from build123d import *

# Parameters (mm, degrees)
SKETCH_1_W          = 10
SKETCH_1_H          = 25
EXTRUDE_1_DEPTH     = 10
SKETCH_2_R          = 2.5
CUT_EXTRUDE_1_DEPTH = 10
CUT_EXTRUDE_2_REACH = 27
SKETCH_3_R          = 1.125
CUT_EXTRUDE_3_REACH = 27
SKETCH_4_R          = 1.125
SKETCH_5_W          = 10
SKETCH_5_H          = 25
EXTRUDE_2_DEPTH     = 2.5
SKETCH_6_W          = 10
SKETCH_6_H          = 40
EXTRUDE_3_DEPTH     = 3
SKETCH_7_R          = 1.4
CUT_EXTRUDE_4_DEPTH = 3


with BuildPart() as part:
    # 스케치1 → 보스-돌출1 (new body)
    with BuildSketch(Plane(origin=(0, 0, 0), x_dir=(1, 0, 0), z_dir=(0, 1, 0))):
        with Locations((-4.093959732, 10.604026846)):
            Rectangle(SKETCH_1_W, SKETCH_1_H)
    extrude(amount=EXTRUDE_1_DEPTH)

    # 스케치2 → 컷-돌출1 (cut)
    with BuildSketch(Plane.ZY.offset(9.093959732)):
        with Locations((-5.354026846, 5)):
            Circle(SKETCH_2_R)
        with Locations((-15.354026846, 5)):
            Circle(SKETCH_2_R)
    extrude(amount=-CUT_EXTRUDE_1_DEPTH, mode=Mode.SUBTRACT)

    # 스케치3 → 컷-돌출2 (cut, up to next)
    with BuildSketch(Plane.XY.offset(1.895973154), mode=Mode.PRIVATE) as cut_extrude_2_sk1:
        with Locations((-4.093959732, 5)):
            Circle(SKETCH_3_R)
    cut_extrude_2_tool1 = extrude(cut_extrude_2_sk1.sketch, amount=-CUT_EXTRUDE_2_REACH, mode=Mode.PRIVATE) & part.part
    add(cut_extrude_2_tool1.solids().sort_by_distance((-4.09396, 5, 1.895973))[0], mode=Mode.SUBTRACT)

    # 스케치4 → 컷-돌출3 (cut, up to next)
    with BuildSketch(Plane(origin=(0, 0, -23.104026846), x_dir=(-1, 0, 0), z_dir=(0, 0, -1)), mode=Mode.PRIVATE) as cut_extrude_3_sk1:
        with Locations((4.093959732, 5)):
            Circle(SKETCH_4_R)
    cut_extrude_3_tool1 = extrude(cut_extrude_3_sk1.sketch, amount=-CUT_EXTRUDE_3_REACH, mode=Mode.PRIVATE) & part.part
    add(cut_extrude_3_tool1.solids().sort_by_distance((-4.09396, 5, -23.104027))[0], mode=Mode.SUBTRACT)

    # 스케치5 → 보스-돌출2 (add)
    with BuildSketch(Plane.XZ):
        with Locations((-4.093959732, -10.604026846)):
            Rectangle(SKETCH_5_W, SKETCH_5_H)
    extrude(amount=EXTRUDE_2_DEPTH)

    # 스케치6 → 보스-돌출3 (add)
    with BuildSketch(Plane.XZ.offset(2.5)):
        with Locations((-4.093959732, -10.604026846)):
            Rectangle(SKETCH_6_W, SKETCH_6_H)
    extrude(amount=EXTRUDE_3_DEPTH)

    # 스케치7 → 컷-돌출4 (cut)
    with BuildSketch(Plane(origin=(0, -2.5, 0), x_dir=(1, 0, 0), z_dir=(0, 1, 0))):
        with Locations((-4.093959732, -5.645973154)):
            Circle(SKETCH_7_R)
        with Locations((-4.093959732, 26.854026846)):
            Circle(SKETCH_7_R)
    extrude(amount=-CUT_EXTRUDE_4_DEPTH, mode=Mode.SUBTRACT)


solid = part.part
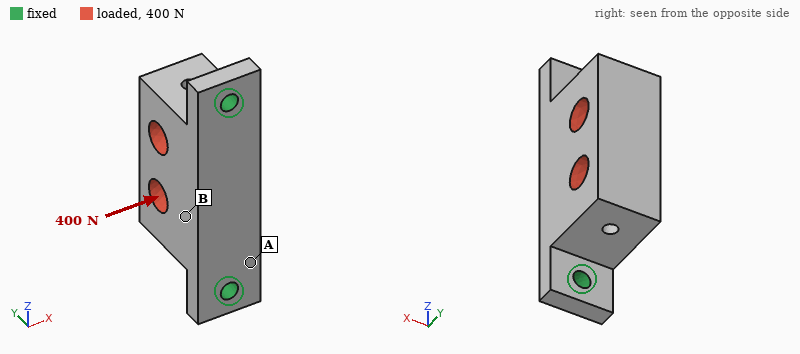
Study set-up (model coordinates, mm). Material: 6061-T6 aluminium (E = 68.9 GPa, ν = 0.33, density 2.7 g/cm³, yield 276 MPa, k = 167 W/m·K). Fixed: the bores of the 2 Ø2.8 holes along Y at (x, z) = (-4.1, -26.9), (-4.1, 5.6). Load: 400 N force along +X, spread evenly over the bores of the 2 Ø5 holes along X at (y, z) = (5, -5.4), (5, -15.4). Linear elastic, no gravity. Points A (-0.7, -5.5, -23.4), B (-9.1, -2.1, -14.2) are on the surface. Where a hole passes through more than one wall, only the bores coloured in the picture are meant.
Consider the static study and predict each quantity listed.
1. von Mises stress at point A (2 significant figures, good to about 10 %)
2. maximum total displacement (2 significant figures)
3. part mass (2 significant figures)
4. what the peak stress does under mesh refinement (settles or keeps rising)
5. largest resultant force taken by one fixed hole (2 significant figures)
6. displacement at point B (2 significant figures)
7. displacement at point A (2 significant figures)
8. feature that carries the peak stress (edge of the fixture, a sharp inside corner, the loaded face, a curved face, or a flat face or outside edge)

38 MPa
53 µm
10 g
keeps rising
200 N
19 µm
8.6 µm
edge of the fixture
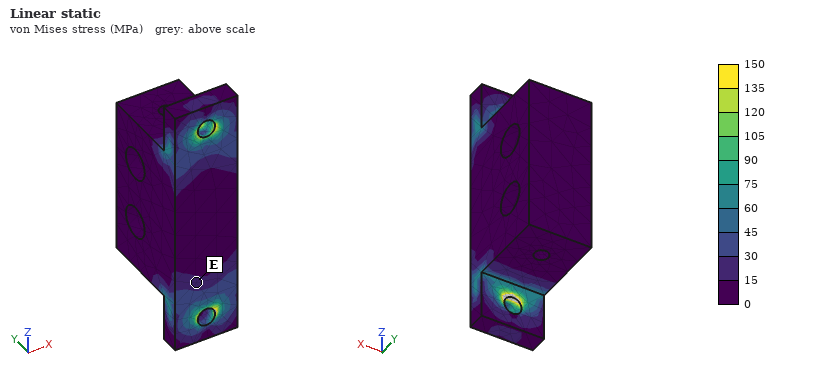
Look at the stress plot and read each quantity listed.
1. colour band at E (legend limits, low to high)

15 to 30 MPa
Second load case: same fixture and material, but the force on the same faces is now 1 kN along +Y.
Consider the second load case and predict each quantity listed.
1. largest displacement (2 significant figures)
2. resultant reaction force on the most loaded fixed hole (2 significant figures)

10 µm
590 N
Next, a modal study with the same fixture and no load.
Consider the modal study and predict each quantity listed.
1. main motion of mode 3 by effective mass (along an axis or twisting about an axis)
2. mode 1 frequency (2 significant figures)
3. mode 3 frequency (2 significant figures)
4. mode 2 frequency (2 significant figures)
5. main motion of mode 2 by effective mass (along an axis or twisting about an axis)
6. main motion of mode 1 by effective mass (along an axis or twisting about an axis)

along Z
6600 Hz
23 kHz
18 kHz
along Y
along X
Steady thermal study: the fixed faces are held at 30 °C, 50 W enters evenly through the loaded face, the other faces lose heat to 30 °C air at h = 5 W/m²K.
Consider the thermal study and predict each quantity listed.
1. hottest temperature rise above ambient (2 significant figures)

46 K
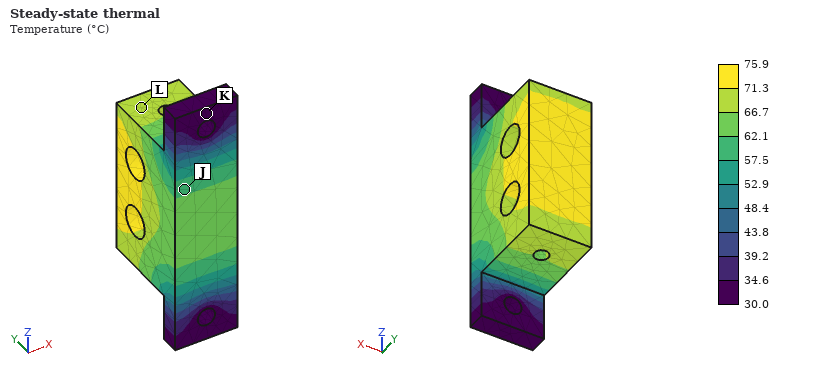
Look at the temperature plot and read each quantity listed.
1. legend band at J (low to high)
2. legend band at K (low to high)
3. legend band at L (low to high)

57.5 to 62.1 °C
30.0 to 34.6 °C
66.7 to 71.3 °C
